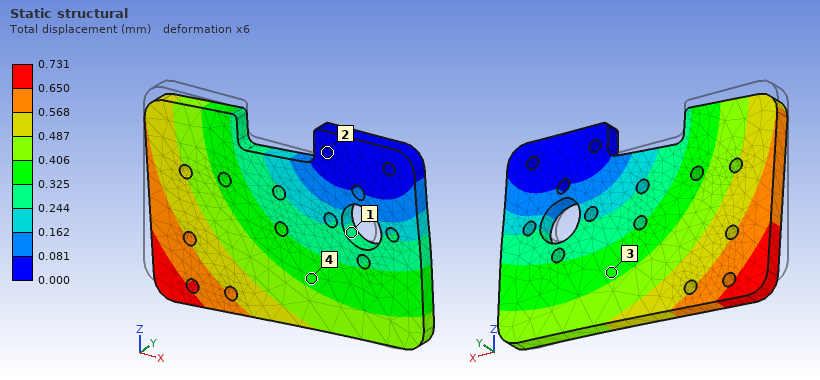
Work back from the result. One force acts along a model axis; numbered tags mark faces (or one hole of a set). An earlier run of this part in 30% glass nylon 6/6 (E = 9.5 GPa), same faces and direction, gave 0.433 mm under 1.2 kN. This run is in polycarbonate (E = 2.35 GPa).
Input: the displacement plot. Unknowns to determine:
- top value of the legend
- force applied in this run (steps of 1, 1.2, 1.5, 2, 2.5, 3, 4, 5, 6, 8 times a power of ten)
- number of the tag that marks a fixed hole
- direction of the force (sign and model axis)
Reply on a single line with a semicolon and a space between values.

0.731 mm; 500 N; 2; +X
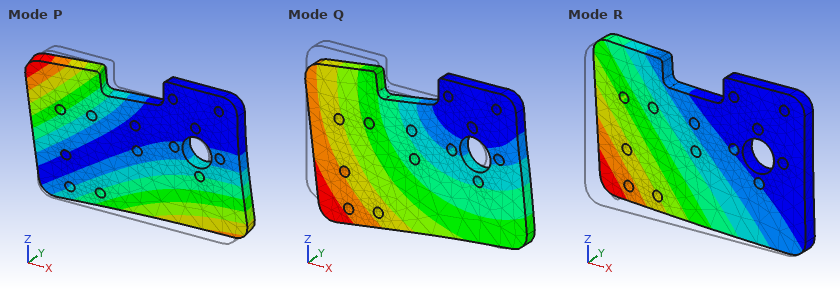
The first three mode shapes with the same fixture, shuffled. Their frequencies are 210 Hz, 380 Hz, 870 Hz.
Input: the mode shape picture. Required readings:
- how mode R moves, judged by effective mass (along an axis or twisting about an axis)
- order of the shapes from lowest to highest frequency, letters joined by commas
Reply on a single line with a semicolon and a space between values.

along Y; R, P, Q
